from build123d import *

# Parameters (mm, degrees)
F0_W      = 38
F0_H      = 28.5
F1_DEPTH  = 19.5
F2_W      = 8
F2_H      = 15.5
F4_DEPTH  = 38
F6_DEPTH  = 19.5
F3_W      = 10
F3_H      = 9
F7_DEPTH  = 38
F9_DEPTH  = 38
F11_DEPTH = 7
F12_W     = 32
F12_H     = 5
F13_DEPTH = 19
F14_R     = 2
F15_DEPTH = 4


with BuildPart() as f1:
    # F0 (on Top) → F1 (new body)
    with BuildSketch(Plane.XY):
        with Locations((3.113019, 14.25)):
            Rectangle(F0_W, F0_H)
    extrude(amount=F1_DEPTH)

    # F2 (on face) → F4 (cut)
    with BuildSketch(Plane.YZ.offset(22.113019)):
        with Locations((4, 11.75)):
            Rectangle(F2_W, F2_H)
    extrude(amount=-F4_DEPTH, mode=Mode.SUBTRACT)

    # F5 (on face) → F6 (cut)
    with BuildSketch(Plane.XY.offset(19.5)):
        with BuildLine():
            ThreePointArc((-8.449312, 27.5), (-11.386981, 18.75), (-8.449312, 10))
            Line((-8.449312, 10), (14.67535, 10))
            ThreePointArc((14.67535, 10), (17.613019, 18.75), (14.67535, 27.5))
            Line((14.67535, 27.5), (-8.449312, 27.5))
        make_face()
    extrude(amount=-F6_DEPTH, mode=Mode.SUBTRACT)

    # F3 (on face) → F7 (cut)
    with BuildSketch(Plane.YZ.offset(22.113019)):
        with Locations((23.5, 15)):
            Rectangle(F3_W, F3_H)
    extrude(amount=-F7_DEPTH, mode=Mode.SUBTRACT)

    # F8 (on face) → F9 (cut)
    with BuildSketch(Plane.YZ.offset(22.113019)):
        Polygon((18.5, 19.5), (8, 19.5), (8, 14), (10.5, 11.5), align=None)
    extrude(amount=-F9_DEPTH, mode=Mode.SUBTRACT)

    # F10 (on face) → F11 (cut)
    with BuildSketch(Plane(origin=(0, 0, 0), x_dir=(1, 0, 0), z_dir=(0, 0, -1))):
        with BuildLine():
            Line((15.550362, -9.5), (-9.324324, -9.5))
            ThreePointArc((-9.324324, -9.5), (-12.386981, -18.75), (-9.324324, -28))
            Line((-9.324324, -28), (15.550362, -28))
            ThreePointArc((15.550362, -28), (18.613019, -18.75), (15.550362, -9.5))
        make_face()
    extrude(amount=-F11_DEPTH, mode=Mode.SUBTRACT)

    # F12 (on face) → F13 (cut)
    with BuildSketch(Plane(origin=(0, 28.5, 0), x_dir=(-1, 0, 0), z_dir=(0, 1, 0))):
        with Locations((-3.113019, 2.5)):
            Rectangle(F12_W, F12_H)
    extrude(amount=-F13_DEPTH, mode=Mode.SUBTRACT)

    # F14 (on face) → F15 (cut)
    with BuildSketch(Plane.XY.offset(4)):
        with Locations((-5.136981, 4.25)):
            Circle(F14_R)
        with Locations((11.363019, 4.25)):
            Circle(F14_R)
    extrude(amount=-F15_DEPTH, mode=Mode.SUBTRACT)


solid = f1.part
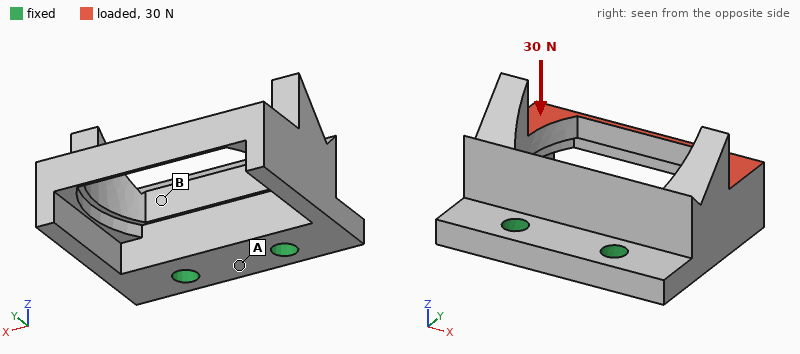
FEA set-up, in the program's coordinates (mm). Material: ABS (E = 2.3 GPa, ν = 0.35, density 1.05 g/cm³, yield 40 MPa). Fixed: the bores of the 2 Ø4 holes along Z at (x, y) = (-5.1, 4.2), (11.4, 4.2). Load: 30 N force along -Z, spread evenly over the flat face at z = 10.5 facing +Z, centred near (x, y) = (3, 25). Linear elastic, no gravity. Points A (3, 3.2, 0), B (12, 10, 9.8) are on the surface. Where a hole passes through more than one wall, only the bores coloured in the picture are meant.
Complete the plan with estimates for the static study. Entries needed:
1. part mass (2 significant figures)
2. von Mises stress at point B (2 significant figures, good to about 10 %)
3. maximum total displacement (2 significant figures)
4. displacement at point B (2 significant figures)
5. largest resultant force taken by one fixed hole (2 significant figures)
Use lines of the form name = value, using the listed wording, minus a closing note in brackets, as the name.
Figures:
part mass = 4.3 g
von Mises stress at point B = 3.0 MPa
maximum total displacement = 0.54 mm
displacement at point B = 0.13 mm
largest resultant force taken by one fixed hole = 20 N
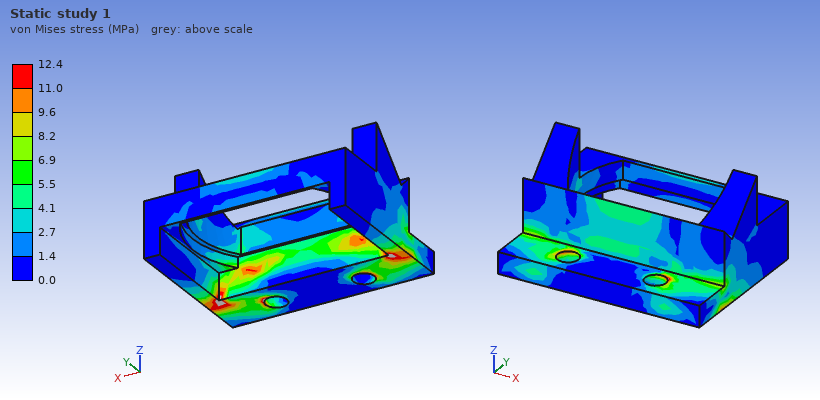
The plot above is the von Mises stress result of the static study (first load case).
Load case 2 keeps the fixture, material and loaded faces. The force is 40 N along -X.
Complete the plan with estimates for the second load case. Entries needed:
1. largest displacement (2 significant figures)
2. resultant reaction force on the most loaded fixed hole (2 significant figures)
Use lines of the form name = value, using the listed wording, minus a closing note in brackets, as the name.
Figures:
largest displacement = 0.51 mm
resultant reaction force on the most loaded fixed hole = 32 N
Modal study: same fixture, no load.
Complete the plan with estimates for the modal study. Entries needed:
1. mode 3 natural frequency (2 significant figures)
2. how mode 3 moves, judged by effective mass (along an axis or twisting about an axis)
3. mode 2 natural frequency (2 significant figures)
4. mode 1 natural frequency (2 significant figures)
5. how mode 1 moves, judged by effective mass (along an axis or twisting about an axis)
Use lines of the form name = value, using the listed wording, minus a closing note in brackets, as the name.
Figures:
mode 3 natural frequency = 1700 Hz
how mode 3 moves, judged by effective mass = along X
mode 2 natural frequency = 1200 Hz
mode 1 natural frequency = 1100 Hz
how mode 1 moves, judged by effective mass = along Z
